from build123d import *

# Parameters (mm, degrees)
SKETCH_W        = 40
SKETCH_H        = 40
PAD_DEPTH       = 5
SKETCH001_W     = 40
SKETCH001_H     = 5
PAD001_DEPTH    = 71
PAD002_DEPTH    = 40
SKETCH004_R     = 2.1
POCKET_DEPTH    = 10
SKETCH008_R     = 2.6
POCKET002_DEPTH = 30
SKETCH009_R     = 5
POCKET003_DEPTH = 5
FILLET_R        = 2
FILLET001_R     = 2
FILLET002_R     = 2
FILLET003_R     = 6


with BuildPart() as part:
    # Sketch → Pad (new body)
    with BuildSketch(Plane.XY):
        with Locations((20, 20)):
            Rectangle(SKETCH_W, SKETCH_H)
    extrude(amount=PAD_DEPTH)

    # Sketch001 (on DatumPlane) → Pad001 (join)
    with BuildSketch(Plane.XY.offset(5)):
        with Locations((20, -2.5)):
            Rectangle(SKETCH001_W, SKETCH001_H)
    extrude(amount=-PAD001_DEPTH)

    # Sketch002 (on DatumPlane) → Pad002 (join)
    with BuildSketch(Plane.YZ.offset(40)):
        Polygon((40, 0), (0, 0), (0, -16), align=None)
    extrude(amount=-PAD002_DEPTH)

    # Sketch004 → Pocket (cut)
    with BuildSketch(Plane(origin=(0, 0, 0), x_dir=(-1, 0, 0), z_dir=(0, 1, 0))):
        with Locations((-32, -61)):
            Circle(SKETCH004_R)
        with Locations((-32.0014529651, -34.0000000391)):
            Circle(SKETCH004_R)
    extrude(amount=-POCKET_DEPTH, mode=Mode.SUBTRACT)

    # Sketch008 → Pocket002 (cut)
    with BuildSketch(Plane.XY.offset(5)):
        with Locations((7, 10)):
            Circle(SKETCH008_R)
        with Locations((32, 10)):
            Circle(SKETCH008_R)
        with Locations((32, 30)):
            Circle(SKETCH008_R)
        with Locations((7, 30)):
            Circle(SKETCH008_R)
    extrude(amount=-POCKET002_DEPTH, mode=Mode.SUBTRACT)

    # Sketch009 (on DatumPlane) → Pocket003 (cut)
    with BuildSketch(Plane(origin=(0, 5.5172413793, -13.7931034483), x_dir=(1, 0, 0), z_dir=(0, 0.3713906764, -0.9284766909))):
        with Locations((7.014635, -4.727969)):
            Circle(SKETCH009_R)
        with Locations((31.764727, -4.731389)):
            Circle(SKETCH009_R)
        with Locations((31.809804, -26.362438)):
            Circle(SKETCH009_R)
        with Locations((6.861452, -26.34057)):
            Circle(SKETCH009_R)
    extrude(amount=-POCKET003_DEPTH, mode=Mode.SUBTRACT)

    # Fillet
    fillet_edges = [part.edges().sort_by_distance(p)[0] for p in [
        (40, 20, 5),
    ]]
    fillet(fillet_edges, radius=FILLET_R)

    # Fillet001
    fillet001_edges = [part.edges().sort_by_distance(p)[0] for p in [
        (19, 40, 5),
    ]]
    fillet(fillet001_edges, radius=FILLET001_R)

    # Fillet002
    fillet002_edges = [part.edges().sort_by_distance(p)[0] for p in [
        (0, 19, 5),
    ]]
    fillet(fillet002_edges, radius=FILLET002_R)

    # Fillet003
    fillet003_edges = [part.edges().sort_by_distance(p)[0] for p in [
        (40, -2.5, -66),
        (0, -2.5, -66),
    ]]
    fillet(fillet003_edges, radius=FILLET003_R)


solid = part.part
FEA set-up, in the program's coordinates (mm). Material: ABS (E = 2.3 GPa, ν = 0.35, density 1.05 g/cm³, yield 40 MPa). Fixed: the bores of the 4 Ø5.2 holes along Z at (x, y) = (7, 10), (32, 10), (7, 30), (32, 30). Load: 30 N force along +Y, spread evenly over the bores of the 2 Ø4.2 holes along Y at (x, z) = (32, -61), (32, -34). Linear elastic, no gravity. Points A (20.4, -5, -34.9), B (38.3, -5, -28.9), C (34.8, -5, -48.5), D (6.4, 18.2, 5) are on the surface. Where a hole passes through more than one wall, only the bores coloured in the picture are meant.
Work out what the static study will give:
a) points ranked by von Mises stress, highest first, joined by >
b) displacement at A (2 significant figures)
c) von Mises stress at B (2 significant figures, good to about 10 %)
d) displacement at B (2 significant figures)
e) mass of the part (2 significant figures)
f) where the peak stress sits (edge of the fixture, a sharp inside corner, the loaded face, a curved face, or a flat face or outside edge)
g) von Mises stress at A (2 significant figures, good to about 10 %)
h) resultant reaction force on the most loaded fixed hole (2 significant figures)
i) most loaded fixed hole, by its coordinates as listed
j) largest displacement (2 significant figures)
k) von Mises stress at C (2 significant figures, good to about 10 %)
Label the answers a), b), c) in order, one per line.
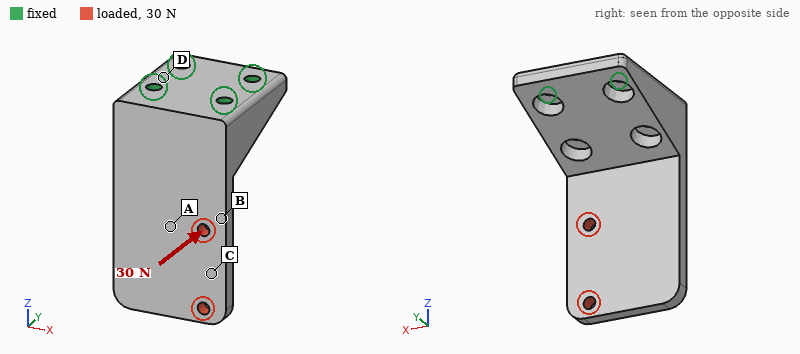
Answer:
a) B > A > C > D
b) 0.23 mm
c) 3.8 MPa
d) 0.17 mm
e) 34 g
f) a flat face or outside edge
g) 2.7 MPa
h) 26 N
i) (32, 10)
j) 0.95 mm
k) 1.6 MPa
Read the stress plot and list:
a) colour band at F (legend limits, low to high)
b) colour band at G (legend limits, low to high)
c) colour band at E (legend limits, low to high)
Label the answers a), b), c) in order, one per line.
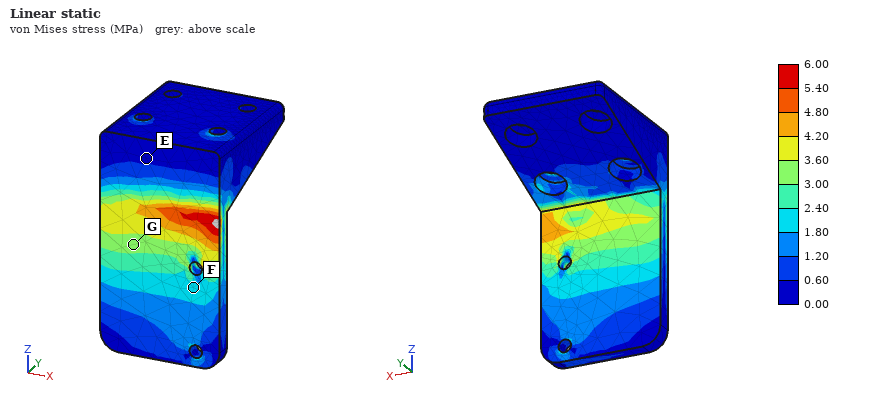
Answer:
a) 1.80 to 2.40 MPa
b) 3.00 to 3.60 MPa
c) 0.00 to 0.60 MPa
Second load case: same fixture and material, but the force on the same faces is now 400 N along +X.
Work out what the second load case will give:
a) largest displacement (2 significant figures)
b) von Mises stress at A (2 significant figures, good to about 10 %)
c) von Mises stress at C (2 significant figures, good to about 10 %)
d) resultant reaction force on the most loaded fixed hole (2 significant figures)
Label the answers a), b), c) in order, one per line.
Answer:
a) 0.61 mm
b) 3.8 MPa
c) 1.9 MPa
d) 650 N
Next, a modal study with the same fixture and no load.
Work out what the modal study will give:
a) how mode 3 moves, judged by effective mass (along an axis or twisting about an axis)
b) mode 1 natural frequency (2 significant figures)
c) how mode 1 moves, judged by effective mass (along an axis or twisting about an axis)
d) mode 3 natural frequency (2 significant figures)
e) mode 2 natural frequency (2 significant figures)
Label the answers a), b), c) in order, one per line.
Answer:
a) along X
b) 430 Hz
c) along Y
d) 1700 Hz
e) 1200 Hz
